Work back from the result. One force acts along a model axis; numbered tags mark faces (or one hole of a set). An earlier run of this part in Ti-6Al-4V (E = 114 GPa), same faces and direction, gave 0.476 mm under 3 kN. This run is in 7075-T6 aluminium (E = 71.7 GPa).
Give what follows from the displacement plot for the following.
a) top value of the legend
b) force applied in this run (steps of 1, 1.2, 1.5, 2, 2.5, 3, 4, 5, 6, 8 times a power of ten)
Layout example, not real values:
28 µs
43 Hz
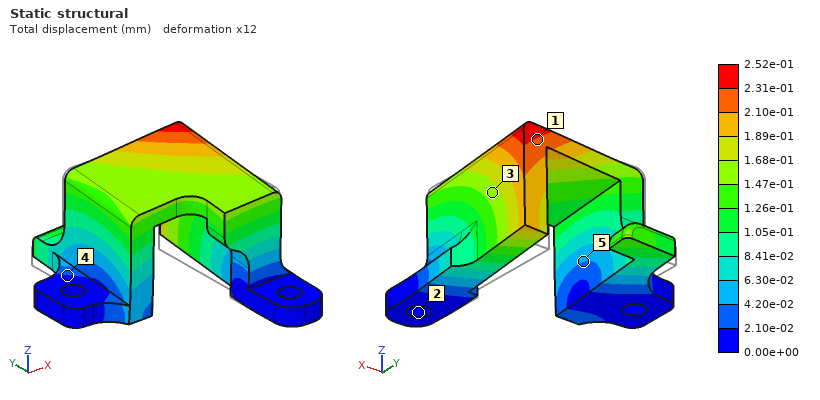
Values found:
2.52e-01 mm
1 kN
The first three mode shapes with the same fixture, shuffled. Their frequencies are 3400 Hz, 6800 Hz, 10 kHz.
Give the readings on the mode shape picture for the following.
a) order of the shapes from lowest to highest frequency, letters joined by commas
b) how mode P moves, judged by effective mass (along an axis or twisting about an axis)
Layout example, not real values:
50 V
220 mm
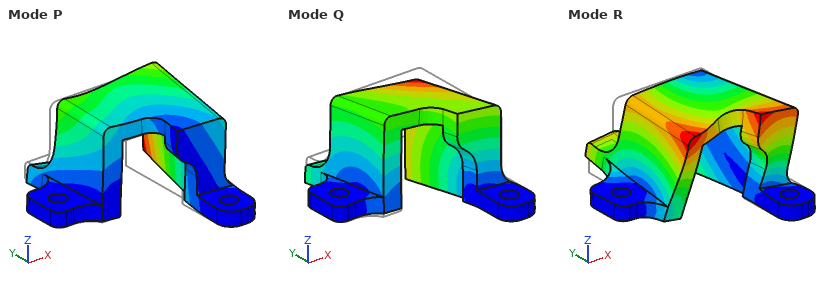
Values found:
Q, P, R
along X
